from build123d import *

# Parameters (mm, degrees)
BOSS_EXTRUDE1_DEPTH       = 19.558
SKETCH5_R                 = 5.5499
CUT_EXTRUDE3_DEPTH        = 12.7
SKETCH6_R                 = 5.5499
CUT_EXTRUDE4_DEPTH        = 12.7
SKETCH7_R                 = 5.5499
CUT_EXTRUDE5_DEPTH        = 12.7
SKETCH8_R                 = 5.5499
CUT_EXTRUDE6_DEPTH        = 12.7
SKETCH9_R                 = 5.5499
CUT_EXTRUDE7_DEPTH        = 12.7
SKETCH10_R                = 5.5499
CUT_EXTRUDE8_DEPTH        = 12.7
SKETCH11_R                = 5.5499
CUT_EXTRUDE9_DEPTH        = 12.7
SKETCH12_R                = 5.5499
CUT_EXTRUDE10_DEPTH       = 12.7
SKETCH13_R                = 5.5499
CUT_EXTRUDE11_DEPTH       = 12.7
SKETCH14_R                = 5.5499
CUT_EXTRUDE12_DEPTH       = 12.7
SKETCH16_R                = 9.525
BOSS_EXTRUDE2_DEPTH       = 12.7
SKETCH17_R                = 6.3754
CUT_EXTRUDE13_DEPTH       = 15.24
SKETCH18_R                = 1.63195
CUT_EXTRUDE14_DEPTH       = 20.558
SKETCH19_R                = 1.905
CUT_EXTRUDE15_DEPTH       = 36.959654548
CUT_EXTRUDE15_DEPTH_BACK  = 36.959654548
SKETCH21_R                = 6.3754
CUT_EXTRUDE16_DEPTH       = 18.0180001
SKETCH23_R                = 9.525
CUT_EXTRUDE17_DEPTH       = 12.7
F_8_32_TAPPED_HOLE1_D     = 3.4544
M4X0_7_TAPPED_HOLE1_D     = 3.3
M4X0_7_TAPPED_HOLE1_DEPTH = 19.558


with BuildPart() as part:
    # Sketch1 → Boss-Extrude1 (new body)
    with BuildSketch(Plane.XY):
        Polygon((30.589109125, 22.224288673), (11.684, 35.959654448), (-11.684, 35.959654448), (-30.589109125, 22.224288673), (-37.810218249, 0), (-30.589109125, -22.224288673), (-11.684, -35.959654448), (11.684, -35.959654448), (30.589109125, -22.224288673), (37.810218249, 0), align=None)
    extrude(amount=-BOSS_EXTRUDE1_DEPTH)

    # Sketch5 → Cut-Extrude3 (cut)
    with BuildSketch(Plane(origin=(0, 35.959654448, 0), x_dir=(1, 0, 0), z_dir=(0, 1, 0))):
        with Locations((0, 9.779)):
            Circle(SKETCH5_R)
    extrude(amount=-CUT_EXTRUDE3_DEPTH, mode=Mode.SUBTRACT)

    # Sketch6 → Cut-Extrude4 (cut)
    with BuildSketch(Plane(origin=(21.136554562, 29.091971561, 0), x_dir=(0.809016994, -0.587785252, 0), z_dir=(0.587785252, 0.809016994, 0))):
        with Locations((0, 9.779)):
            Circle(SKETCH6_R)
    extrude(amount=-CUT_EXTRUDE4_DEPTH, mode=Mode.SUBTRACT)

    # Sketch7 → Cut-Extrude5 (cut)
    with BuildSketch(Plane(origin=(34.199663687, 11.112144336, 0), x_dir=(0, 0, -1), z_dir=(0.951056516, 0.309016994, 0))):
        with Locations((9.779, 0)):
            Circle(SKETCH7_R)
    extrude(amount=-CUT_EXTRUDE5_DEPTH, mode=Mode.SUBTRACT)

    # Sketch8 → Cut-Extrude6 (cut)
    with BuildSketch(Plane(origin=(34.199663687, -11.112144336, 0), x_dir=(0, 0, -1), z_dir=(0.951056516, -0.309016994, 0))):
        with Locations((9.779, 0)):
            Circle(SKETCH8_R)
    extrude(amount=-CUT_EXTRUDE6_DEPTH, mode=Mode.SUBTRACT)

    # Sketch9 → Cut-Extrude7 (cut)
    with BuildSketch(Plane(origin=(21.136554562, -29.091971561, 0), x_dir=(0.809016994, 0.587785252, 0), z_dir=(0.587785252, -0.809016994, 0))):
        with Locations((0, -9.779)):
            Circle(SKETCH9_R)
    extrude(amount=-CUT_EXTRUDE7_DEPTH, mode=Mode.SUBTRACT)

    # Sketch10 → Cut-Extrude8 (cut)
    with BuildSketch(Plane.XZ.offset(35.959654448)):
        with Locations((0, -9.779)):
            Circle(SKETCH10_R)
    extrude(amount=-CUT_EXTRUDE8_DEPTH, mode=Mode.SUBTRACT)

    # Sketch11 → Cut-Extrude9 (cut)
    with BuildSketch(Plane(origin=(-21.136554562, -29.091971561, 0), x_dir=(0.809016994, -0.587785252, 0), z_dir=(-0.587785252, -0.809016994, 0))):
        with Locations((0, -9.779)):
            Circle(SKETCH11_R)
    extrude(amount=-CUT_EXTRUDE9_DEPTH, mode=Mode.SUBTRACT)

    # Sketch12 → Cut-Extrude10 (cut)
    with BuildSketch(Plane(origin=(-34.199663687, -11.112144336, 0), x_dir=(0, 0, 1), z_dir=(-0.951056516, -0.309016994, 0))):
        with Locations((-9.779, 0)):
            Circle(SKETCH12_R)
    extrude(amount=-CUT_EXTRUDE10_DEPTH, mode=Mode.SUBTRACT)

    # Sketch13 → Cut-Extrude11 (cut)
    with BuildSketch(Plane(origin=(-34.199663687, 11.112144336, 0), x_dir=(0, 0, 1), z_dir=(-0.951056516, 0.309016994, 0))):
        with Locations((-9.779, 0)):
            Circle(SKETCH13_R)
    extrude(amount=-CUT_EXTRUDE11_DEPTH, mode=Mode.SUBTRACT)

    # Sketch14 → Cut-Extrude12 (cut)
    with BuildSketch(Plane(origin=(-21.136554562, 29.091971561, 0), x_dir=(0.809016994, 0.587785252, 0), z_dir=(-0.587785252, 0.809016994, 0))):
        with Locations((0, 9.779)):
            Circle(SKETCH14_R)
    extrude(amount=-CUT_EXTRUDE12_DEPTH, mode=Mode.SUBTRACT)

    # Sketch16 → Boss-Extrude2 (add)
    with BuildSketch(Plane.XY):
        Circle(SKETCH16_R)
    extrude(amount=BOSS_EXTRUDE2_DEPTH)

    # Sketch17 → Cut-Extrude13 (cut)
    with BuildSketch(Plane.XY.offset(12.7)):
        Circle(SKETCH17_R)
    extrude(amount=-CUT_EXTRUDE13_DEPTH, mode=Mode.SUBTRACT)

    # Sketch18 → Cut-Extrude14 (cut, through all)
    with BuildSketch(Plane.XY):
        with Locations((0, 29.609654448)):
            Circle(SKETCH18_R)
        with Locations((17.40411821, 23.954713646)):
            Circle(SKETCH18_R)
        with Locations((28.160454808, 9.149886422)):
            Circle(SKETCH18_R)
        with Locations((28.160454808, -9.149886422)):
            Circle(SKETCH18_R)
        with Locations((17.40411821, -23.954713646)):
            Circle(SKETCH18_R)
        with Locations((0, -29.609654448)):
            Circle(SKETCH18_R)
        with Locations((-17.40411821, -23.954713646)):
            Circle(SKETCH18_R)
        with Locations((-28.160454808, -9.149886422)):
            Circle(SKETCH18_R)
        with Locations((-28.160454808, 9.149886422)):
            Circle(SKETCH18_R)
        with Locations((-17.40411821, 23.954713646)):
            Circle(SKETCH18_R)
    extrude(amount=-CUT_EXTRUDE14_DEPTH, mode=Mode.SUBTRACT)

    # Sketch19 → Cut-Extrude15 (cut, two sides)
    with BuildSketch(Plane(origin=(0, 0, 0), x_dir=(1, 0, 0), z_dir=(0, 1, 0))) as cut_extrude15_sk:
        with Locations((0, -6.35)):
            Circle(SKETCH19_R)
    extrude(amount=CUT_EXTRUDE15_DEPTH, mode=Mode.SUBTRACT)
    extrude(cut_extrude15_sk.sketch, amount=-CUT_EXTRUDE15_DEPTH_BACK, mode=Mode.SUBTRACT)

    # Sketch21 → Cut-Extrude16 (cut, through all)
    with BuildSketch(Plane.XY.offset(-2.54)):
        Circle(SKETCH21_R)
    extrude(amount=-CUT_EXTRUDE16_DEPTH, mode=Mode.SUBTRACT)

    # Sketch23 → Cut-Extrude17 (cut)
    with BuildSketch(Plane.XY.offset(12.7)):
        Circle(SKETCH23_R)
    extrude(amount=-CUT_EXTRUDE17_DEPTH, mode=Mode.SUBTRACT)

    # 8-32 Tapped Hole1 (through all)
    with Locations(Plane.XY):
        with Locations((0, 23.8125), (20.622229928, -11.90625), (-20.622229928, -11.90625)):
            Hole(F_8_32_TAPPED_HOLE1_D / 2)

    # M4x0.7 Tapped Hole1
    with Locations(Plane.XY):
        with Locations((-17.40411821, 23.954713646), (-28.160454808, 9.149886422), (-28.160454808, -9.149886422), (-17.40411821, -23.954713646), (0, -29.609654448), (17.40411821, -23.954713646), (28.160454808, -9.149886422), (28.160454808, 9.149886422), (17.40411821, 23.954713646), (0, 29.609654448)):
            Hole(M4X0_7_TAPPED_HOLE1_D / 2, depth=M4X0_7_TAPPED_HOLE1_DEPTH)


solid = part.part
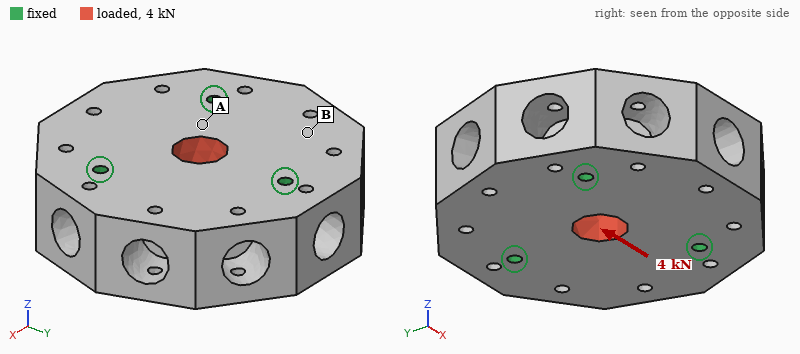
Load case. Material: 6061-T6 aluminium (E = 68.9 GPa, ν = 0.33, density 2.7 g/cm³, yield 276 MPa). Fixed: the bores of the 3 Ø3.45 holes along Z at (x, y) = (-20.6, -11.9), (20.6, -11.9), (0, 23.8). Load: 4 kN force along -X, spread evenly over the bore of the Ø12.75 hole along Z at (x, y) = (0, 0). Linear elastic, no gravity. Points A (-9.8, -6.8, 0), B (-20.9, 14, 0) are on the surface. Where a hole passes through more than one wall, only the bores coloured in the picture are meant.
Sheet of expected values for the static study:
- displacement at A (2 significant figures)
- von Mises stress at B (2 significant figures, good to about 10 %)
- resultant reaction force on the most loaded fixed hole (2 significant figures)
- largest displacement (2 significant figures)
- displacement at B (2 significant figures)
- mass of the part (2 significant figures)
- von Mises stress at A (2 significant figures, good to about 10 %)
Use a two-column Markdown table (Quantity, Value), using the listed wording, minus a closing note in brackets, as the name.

| Quantity | Value |
|---|---|
| displacement at A | 1.1 µm |
| von Mises stress at B | 2.3 MPa |
| resultant reaction force on the most loaded fixed hole | 1.4 kN |
| largest displacement | 2.2 µm |
| displacement at B | 1.3 µm |
| mass of the part | 180 g |
| von Mises stress at A | 5.3 MPa |
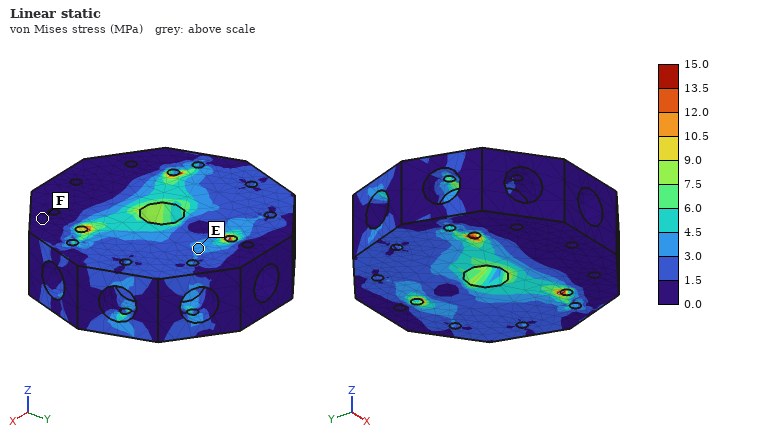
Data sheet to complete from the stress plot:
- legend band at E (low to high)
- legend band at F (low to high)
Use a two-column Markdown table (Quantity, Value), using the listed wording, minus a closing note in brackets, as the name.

| Quantity | Value |
|---|---|
| legend band at E | 3.0 to 4.5 MPa |
| legend band at F | 0.0 to 1.5 MPa |
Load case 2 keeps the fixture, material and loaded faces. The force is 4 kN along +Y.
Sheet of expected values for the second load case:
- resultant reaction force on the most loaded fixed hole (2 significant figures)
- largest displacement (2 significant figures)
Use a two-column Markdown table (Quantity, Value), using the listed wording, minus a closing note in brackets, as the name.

| Quantity | Value |
|---|---|
| resultant reaction force on the most loaded fixed hole | 1.4 kN |
| largest displacement | 2.3 µm |
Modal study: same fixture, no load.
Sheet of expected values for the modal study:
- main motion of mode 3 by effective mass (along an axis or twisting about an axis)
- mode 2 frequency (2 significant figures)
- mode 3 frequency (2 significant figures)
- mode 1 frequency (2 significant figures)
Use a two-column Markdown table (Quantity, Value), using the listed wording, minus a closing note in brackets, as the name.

| Quantity | Value |
|---|---|
| main motion of mode 3 by effective mass | along Z |
| mode 2 frequency | 14 kHz |
| mode 3 frequency | 17 kHz |
| mode 1 frequency | 14 kHz |
